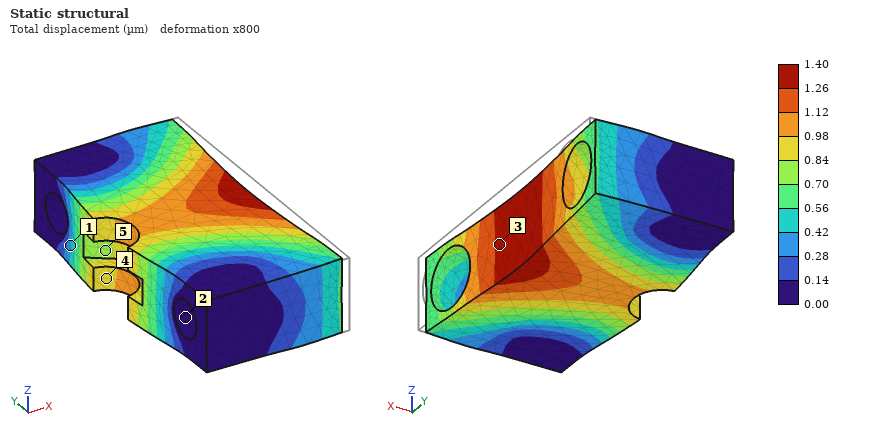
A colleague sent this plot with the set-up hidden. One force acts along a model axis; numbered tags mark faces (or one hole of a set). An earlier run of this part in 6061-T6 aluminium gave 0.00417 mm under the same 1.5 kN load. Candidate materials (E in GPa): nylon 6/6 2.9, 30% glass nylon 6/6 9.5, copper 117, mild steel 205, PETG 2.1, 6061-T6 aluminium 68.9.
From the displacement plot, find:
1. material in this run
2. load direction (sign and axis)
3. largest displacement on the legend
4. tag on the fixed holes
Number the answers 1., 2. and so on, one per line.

1. mild steel
2. -X
3. 1.40 µm
4. 2
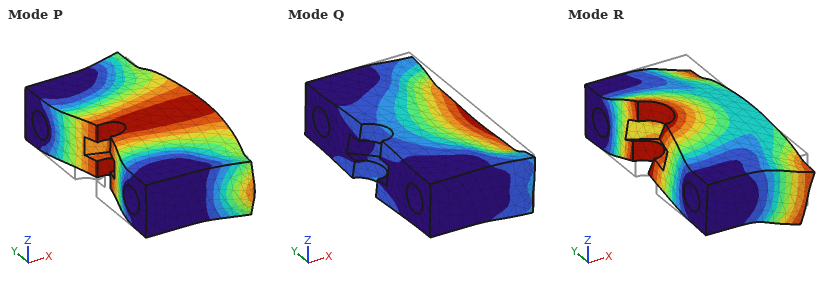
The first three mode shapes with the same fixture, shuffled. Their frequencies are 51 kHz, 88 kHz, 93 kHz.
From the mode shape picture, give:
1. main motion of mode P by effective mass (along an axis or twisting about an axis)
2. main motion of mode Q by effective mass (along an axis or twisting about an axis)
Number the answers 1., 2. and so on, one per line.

1. along X
2. along Z
